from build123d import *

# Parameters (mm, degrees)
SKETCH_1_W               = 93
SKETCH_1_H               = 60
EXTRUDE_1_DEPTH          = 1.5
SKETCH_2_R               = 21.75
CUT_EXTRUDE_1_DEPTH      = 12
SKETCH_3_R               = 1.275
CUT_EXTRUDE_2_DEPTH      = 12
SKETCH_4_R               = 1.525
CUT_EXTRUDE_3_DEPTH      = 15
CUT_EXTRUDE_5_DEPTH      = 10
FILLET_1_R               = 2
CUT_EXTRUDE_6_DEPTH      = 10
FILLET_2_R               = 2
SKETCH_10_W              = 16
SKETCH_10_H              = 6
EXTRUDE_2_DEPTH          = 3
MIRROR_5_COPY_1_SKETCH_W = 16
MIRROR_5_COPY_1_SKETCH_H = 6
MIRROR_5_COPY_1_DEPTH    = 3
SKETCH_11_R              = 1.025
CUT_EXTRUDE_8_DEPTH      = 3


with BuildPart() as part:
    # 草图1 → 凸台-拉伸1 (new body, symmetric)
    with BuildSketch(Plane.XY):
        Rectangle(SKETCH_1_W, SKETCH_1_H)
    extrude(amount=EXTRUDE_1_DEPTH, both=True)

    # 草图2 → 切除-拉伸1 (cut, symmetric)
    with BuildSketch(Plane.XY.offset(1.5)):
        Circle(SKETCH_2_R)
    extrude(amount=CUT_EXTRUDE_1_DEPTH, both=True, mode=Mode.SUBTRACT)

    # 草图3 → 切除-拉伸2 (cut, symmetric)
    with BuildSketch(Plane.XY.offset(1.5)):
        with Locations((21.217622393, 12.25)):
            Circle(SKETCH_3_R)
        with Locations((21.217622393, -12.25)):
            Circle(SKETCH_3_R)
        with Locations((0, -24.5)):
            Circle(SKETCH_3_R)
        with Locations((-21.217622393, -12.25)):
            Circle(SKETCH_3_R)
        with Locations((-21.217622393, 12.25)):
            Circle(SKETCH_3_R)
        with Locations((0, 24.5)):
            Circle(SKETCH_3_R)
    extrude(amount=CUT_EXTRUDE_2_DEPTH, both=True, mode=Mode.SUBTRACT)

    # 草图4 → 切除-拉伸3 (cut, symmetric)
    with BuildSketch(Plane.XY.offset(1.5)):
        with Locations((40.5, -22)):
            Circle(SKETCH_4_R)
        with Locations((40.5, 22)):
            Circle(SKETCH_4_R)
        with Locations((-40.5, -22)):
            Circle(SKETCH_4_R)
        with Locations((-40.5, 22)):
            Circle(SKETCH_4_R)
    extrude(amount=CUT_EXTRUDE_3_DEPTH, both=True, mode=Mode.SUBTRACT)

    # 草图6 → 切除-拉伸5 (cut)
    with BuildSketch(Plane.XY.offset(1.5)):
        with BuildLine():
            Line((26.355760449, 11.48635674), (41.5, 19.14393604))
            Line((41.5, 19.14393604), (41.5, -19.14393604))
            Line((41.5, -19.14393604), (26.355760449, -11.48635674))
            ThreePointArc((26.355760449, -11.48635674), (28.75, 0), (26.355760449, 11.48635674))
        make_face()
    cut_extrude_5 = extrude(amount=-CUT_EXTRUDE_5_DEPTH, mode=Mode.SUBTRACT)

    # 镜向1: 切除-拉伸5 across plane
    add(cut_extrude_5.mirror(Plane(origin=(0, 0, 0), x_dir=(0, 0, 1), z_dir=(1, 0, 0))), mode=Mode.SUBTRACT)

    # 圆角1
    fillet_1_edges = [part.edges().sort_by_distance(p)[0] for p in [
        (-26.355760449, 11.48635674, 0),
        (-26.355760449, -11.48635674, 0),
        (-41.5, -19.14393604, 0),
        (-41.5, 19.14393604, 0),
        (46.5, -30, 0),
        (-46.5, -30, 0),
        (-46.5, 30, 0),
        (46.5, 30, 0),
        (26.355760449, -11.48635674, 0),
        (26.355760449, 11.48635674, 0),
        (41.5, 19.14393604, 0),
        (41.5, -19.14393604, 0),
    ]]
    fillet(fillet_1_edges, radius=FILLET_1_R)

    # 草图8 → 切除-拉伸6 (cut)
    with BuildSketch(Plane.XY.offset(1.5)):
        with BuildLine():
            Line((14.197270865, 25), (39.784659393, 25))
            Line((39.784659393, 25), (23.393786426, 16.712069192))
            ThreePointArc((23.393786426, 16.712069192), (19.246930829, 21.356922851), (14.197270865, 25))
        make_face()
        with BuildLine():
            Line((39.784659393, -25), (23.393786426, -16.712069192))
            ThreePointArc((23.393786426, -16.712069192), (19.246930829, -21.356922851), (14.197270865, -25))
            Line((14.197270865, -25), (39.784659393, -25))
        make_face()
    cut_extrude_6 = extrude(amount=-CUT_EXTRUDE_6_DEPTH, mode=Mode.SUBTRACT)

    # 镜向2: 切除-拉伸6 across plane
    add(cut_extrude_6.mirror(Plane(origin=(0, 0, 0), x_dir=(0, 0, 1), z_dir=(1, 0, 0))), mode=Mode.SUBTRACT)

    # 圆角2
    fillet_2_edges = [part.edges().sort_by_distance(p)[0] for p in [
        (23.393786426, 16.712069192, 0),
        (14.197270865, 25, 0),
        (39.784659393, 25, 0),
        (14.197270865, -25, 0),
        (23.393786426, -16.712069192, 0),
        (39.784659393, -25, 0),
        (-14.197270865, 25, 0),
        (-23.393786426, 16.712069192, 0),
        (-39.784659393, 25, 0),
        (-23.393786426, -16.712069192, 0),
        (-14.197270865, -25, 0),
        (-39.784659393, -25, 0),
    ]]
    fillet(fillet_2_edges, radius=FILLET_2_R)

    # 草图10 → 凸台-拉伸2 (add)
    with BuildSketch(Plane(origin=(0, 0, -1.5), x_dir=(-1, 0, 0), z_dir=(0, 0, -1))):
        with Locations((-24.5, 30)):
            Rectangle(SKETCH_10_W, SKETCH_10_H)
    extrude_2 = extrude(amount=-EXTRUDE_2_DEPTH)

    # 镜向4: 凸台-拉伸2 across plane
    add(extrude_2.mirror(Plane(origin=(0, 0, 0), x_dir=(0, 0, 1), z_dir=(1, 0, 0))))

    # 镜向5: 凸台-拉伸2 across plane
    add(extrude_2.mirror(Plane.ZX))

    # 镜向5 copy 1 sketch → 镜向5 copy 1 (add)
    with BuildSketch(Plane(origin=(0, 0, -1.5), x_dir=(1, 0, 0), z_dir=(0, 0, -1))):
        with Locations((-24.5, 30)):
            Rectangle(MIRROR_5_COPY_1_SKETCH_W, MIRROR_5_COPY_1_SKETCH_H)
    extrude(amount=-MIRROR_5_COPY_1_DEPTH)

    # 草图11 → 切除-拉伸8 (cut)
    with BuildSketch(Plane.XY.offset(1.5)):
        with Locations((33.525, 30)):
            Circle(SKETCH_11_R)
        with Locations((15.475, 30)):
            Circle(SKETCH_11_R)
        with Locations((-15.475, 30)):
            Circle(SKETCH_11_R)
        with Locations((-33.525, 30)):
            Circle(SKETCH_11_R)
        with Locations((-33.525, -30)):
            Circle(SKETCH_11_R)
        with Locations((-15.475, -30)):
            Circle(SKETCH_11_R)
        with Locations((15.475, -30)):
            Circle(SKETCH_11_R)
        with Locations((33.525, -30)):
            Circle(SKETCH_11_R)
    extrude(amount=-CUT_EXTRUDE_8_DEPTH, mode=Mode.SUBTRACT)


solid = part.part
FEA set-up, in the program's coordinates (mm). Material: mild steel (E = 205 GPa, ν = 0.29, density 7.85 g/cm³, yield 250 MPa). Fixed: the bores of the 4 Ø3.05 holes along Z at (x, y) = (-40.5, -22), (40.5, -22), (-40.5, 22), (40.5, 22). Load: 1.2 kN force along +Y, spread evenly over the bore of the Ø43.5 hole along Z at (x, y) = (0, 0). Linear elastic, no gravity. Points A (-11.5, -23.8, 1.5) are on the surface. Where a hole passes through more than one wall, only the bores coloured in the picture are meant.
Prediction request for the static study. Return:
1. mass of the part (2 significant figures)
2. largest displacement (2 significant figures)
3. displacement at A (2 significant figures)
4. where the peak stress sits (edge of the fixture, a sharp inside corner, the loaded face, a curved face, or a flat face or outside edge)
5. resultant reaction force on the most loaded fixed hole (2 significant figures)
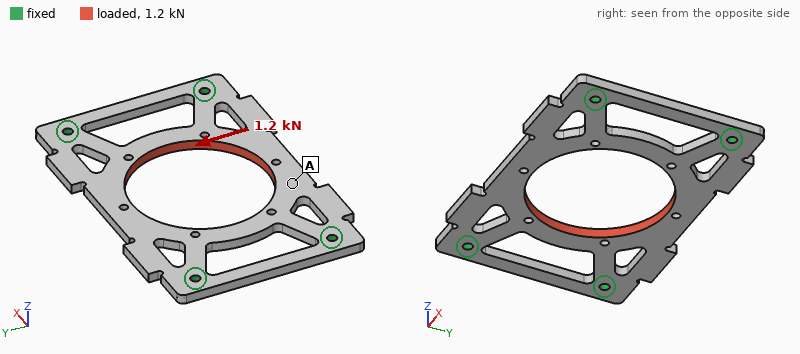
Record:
72 g
16 µm
14 µm
a curved face
310 N
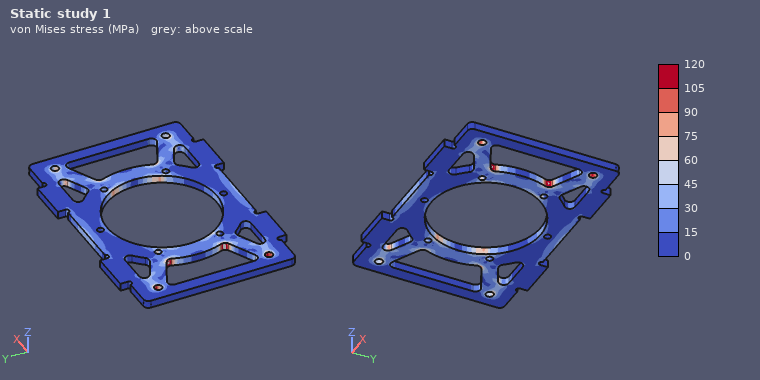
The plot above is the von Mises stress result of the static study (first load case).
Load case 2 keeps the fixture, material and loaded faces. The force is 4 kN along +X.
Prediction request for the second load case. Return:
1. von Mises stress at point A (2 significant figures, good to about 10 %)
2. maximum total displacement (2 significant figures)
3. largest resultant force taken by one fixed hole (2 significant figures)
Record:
13 MPa
8.8 µm
1.0 kN
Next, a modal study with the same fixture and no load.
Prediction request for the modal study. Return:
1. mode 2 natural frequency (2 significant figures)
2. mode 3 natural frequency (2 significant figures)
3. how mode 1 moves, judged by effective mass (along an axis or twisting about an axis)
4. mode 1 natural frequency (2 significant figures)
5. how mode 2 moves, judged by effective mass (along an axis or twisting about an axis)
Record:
2600 Hz
4800 Hz
along Z
2300 Hz
twisting about X
